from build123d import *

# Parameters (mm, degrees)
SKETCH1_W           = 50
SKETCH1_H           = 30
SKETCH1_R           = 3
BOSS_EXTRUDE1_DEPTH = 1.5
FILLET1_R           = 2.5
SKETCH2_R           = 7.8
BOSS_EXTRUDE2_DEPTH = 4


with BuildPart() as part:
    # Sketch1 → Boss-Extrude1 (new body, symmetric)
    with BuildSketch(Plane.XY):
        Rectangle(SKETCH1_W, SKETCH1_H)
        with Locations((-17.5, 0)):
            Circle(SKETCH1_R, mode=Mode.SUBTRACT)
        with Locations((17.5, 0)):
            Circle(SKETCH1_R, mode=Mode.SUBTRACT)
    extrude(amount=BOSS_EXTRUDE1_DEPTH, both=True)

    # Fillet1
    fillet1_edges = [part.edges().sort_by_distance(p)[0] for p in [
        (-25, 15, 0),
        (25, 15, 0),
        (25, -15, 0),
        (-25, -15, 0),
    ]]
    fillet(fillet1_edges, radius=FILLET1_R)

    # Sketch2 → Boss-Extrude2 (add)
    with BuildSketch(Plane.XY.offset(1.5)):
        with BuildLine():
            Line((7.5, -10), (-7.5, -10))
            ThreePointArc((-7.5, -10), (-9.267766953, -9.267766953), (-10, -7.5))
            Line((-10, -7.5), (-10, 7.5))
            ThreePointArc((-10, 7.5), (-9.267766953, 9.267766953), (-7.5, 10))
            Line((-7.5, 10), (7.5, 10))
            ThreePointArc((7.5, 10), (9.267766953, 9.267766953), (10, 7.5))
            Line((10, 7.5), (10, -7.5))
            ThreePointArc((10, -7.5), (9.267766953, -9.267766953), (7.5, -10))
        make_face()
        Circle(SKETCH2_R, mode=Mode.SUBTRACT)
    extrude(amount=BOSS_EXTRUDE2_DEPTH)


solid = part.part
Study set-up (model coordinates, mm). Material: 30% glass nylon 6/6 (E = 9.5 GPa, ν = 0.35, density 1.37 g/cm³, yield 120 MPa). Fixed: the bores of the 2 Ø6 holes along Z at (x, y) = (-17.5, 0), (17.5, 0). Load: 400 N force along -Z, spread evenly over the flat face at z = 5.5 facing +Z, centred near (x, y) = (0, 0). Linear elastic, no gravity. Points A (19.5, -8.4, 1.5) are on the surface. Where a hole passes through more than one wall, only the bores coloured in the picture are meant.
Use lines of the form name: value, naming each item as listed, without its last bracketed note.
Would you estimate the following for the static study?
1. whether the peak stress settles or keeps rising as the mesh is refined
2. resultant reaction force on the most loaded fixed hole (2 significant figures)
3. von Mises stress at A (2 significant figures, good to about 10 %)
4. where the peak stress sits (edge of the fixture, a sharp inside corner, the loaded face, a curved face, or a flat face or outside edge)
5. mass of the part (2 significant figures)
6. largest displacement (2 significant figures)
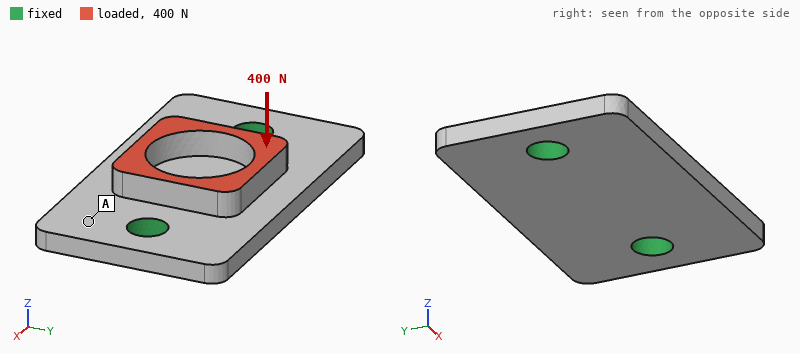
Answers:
whether the peak stress settles or keeps rising as the mesh is refined: keeps rising
resultant reaction force on the most loaded fixed hole: 210 N
von Mises stress at A: 4.9 MPa
where the peak stress sits: edge of the fixture
mass of the part: 7.0 g
largest displacement: 72 µm
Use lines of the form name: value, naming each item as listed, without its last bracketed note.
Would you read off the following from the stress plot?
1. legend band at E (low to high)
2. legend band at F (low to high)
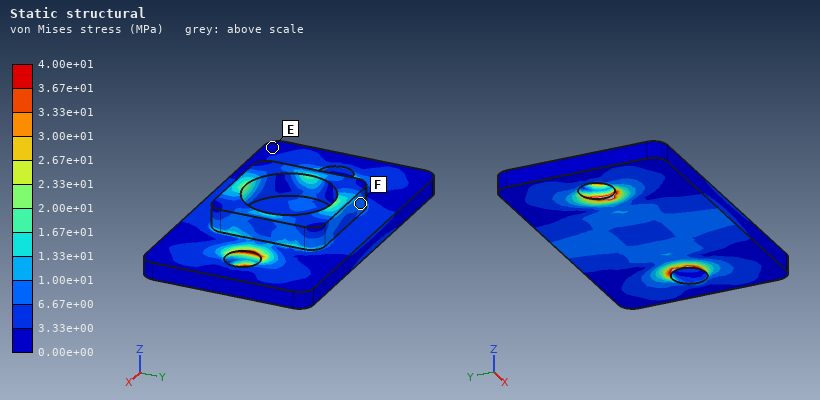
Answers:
legend band at E: 0.00e+00 to 3.33e+00 MPa
legend band at F: 6.67e+00 to 1.00e+01 MPa
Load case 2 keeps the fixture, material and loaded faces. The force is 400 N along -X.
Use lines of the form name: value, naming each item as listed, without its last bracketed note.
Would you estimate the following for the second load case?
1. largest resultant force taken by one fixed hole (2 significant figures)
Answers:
largest resultant force taken by one fixed hole: 220 N
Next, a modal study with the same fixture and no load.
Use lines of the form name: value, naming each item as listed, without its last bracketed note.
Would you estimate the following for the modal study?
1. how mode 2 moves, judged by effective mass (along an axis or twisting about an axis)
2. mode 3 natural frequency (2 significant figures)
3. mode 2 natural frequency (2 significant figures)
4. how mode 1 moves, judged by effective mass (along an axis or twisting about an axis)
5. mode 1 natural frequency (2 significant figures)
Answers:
how mode 2 moves, judged by effective mass: along Z
mode 3 natural frequency: 8500 Hz
mode 2 natural frequency: 6500 Hz
how mode 1 moves, judged by effective mass: twisting about X
mode 1 natural frequency: 4800 Hz
